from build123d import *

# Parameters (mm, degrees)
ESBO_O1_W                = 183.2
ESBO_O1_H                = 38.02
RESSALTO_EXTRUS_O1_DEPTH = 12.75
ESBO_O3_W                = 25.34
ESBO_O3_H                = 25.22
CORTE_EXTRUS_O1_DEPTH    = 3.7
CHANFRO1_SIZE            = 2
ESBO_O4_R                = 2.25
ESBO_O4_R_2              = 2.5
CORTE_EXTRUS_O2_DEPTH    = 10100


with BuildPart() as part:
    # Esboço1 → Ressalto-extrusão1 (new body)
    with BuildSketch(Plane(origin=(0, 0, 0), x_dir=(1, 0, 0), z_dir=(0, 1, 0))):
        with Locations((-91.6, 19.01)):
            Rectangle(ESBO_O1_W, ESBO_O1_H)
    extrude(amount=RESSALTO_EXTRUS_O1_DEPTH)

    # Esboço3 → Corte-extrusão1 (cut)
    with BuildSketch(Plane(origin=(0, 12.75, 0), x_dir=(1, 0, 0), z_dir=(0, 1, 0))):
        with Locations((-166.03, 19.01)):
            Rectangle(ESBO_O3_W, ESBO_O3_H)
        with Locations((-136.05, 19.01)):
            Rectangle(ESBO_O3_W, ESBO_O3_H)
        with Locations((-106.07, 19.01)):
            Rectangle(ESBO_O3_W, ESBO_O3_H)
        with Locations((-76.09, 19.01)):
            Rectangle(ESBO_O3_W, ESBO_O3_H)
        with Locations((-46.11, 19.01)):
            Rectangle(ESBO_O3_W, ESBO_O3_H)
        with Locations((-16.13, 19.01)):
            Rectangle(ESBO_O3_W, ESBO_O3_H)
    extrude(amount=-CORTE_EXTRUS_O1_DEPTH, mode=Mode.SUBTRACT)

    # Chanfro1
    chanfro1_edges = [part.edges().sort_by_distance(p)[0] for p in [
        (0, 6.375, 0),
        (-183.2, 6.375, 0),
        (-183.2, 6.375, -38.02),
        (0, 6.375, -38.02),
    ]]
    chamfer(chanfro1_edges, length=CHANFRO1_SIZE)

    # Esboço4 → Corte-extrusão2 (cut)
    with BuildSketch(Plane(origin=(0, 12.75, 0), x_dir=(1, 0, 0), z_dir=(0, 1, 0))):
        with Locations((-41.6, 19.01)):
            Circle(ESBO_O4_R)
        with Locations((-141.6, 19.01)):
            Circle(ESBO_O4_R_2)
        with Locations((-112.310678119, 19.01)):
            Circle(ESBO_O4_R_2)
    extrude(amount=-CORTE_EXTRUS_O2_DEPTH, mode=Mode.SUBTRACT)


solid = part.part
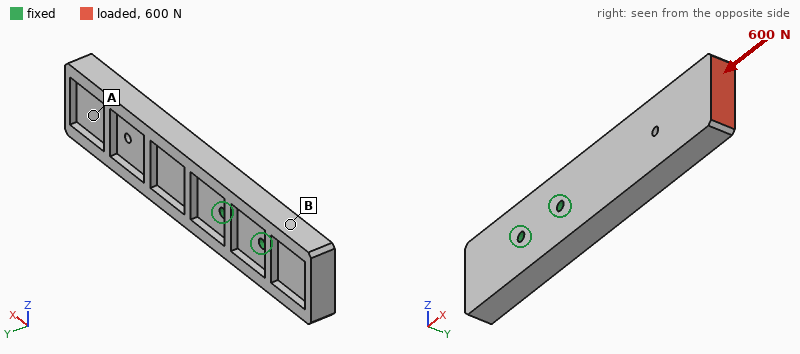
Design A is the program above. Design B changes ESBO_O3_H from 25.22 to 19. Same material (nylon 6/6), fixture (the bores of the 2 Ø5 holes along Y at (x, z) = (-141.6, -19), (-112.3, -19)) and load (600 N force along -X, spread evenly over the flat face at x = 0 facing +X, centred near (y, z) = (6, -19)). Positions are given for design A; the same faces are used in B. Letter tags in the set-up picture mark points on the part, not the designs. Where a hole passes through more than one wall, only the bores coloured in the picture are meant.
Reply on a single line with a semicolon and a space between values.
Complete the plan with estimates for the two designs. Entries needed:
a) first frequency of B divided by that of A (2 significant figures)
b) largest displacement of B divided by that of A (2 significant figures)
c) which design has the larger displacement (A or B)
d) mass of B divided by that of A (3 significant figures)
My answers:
1.0; 0.69; A; 1.05
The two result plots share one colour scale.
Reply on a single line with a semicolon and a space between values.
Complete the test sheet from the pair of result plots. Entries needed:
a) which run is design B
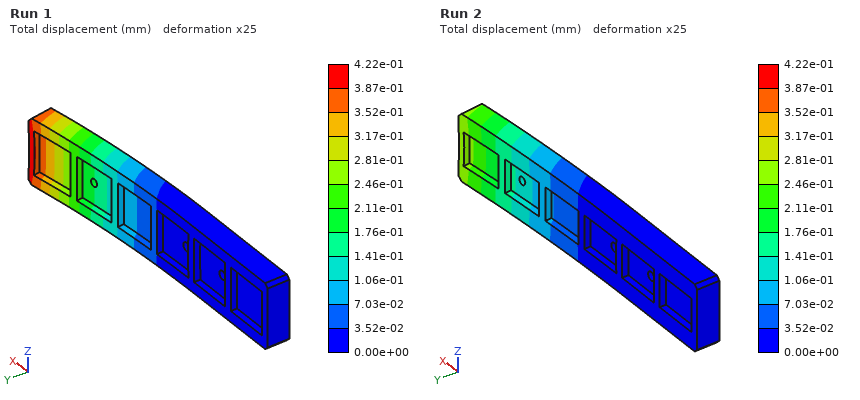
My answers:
Run 2
